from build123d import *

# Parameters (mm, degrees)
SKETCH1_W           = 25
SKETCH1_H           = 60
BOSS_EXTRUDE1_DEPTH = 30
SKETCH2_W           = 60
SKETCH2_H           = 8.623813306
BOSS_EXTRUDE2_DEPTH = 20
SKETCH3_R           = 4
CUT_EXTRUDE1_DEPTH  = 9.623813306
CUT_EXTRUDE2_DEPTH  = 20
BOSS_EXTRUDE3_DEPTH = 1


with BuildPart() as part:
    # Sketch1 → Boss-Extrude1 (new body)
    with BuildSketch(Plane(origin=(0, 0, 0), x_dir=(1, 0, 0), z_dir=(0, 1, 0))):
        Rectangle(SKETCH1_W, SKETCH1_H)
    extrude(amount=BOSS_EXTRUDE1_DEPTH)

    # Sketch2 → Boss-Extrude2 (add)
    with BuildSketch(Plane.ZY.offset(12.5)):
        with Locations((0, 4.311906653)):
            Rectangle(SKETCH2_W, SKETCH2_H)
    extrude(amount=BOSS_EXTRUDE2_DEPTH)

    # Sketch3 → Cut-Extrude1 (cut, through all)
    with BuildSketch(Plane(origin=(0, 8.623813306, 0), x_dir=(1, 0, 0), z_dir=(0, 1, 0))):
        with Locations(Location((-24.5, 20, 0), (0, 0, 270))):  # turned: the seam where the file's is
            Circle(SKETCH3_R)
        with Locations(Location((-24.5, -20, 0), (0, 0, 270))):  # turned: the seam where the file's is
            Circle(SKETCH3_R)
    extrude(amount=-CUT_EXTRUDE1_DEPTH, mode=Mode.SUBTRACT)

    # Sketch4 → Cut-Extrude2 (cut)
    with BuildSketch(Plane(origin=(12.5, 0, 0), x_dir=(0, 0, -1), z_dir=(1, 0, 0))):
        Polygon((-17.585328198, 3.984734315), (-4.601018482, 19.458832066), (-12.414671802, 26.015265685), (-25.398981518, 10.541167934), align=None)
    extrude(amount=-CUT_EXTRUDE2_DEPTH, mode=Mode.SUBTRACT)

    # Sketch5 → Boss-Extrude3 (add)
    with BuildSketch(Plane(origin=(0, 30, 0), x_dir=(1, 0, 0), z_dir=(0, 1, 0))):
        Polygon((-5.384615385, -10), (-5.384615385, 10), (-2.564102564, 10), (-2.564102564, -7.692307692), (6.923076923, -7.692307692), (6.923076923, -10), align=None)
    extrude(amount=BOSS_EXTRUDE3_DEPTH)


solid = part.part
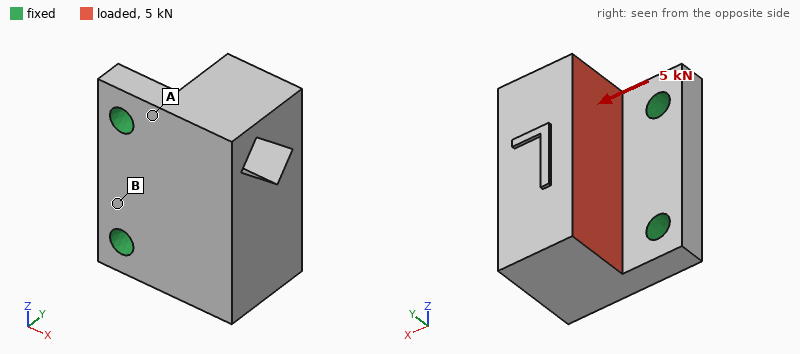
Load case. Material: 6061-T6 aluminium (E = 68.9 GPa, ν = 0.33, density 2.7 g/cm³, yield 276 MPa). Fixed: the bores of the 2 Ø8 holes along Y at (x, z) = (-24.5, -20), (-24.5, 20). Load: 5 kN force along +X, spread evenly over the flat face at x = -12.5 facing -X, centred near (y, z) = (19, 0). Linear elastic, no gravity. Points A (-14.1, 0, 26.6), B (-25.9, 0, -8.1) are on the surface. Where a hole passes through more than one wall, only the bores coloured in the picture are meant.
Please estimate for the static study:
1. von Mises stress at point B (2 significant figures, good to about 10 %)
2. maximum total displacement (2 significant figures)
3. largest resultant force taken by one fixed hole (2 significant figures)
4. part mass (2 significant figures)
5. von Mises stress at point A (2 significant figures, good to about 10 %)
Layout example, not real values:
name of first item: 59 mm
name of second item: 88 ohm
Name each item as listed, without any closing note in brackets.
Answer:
von Mises stress at point B: 26 MPa
maximum total displacement: 0.21 mm
largest resultant force taken by one fixed hole: 2.5 kN
part mass: 140 g
von Mises stress at point A: 85 MPa
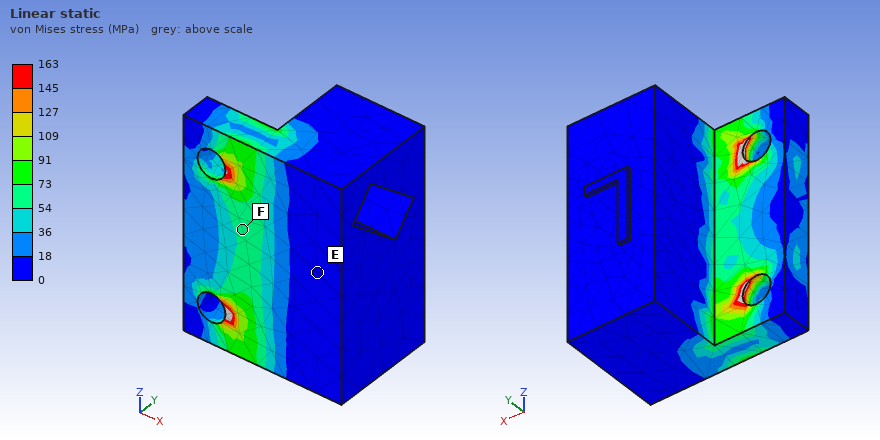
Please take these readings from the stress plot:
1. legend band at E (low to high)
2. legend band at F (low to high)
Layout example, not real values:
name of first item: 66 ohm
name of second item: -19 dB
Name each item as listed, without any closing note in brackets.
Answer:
legend band at E: 0 to 18 MPa
legend band at F: 54 to 73 MPa
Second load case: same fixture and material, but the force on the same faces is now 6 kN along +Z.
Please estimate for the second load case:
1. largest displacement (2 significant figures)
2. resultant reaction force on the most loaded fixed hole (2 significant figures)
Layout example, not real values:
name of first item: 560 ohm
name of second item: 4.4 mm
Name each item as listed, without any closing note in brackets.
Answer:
largest displacement: 44 µm
resultant reaction force on the most loaded fixed hole: 3.9 kN
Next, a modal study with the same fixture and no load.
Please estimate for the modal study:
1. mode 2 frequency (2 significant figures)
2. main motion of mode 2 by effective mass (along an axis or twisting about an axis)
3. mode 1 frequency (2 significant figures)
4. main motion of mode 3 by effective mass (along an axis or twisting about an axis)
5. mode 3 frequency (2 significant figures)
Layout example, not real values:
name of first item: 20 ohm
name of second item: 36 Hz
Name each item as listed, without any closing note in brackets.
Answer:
mode 2 frequency: 6800 Hz
main motion of mode 2 by effective mass: along Z
mode 1 frequency: 2500 Hz
main motion of mode 3 by effective mass: along Z
mode 3 frequency: 9800 Hz
